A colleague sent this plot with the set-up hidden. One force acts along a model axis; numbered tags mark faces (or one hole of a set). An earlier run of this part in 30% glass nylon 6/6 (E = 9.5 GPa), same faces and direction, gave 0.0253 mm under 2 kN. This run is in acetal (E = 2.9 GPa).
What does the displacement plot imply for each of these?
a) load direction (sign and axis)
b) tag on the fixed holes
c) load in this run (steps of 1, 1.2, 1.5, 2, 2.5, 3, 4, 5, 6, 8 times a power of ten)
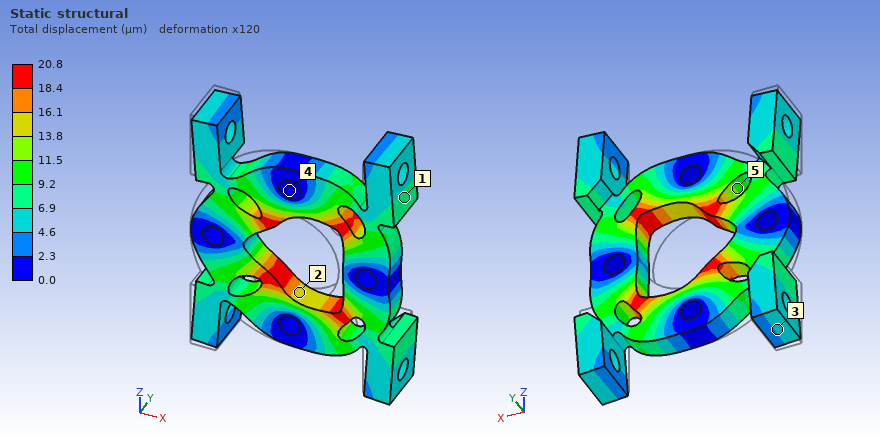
+X
4
500 N
